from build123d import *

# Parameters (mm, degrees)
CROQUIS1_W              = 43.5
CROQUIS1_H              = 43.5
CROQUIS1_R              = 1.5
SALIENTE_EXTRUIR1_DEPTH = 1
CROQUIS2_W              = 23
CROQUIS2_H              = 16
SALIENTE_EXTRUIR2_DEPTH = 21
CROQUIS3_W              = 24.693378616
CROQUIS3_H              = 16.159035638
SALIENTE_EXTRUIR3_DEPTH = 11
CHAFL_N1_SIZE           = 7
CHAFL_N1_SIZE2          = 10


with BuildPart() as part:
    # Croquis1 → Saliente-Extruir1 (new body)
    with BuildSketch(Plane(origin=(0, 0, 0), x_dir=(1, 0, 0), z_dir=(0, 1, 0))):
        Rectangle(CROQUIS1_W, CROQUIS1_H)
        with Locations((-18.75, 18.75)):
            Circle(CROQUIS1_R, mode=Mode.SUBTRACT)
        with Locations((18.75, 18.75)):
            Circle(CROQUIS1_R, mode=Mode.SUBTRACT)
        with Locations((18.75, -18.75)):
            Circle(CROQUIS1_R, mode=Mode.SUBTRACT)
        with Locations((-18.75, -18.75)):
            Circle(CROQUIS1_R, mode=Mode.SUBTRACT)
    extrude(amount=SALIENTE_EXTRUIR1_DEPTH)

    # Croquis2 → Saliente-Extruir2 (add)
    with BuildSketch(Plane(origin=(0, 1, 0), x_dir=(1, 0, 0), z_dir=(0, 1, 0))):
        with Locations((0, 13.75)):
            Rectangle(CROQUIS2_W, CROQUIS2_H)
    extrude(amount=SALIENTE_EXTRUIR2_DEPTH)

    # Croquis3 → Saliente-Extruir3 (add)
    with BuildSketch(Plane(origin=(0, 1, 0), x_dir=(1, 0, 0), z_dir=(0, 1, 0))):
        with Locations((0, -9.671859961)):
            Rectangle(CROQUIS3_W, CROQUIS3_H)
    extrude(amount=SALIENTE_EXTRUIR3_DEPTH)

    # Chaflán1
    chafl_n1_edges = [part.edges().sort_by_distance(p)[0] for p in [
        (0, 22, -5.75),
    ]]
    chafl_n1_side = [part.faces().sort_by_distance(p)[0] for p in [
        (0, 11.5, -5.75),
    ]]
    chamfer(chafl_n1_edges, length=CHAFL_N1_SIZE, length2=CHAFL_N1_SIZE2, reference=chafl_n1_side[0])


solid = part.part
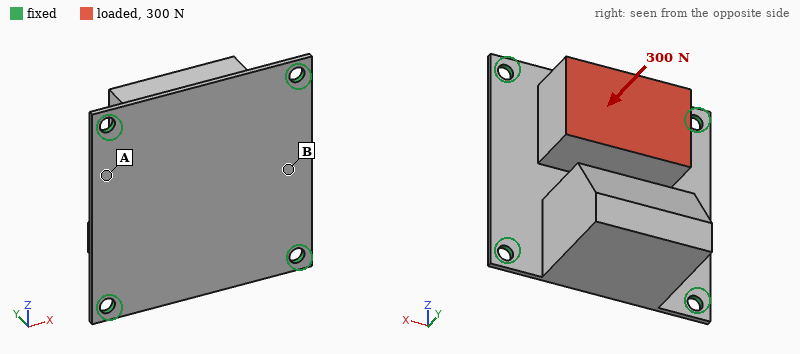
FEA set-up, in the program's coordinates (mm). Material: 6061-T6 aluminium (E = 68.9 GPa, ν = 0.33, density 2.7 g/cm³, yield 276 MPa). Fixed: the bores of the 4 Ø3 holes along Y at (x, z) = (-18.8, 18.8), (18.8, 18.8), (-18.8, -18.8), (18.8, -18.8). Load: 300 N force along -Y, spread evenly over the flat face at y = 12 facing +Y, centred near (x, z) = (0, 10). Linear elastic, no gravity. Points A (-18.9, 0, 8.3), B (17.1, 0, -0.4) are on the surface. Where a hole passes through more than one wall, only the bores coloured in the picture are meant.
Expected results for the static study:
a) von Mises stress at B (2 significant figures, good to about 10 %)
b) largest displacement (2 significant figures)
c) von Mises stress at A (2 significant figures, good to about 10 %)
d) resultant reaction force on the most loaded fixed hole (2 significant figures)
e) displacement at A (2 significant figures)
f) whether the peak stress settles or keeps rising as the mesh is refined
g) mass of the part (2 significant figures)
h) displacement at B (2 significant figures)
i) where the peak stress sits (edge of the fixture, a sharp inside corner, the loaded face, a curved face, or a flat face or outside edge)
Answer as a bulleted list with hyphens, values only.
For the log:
- 63 MPa
- 0.23 mm
- 30 MPa
- 130 N
- 0.093 mm
- keeps rising
- 36 g
- 0.15 mm
- edge of the fixture
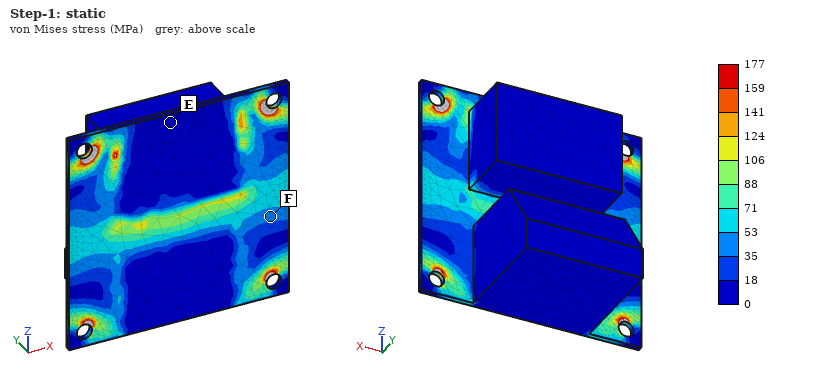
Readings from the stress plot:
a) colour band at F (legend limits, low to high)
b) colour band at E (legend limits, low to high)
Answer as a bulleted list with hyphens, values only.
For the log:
- 35 to 53 MPa
- 0 to 18 MPa
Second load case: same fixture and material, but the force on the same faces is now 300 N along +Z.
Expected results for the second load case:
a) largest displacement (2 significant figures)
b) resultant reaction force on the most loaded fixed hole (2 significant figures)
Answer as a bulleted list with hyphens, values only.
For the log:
- 0.30 mm
- 110 N
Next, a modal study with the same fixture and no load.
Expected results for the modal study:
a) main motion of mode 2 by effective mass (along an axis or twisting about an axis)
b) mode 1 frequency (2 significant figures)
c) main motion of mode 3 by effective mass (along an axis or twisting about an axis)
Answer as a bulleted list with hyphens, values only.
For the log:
- along Y
- 990 Hz
- along X
